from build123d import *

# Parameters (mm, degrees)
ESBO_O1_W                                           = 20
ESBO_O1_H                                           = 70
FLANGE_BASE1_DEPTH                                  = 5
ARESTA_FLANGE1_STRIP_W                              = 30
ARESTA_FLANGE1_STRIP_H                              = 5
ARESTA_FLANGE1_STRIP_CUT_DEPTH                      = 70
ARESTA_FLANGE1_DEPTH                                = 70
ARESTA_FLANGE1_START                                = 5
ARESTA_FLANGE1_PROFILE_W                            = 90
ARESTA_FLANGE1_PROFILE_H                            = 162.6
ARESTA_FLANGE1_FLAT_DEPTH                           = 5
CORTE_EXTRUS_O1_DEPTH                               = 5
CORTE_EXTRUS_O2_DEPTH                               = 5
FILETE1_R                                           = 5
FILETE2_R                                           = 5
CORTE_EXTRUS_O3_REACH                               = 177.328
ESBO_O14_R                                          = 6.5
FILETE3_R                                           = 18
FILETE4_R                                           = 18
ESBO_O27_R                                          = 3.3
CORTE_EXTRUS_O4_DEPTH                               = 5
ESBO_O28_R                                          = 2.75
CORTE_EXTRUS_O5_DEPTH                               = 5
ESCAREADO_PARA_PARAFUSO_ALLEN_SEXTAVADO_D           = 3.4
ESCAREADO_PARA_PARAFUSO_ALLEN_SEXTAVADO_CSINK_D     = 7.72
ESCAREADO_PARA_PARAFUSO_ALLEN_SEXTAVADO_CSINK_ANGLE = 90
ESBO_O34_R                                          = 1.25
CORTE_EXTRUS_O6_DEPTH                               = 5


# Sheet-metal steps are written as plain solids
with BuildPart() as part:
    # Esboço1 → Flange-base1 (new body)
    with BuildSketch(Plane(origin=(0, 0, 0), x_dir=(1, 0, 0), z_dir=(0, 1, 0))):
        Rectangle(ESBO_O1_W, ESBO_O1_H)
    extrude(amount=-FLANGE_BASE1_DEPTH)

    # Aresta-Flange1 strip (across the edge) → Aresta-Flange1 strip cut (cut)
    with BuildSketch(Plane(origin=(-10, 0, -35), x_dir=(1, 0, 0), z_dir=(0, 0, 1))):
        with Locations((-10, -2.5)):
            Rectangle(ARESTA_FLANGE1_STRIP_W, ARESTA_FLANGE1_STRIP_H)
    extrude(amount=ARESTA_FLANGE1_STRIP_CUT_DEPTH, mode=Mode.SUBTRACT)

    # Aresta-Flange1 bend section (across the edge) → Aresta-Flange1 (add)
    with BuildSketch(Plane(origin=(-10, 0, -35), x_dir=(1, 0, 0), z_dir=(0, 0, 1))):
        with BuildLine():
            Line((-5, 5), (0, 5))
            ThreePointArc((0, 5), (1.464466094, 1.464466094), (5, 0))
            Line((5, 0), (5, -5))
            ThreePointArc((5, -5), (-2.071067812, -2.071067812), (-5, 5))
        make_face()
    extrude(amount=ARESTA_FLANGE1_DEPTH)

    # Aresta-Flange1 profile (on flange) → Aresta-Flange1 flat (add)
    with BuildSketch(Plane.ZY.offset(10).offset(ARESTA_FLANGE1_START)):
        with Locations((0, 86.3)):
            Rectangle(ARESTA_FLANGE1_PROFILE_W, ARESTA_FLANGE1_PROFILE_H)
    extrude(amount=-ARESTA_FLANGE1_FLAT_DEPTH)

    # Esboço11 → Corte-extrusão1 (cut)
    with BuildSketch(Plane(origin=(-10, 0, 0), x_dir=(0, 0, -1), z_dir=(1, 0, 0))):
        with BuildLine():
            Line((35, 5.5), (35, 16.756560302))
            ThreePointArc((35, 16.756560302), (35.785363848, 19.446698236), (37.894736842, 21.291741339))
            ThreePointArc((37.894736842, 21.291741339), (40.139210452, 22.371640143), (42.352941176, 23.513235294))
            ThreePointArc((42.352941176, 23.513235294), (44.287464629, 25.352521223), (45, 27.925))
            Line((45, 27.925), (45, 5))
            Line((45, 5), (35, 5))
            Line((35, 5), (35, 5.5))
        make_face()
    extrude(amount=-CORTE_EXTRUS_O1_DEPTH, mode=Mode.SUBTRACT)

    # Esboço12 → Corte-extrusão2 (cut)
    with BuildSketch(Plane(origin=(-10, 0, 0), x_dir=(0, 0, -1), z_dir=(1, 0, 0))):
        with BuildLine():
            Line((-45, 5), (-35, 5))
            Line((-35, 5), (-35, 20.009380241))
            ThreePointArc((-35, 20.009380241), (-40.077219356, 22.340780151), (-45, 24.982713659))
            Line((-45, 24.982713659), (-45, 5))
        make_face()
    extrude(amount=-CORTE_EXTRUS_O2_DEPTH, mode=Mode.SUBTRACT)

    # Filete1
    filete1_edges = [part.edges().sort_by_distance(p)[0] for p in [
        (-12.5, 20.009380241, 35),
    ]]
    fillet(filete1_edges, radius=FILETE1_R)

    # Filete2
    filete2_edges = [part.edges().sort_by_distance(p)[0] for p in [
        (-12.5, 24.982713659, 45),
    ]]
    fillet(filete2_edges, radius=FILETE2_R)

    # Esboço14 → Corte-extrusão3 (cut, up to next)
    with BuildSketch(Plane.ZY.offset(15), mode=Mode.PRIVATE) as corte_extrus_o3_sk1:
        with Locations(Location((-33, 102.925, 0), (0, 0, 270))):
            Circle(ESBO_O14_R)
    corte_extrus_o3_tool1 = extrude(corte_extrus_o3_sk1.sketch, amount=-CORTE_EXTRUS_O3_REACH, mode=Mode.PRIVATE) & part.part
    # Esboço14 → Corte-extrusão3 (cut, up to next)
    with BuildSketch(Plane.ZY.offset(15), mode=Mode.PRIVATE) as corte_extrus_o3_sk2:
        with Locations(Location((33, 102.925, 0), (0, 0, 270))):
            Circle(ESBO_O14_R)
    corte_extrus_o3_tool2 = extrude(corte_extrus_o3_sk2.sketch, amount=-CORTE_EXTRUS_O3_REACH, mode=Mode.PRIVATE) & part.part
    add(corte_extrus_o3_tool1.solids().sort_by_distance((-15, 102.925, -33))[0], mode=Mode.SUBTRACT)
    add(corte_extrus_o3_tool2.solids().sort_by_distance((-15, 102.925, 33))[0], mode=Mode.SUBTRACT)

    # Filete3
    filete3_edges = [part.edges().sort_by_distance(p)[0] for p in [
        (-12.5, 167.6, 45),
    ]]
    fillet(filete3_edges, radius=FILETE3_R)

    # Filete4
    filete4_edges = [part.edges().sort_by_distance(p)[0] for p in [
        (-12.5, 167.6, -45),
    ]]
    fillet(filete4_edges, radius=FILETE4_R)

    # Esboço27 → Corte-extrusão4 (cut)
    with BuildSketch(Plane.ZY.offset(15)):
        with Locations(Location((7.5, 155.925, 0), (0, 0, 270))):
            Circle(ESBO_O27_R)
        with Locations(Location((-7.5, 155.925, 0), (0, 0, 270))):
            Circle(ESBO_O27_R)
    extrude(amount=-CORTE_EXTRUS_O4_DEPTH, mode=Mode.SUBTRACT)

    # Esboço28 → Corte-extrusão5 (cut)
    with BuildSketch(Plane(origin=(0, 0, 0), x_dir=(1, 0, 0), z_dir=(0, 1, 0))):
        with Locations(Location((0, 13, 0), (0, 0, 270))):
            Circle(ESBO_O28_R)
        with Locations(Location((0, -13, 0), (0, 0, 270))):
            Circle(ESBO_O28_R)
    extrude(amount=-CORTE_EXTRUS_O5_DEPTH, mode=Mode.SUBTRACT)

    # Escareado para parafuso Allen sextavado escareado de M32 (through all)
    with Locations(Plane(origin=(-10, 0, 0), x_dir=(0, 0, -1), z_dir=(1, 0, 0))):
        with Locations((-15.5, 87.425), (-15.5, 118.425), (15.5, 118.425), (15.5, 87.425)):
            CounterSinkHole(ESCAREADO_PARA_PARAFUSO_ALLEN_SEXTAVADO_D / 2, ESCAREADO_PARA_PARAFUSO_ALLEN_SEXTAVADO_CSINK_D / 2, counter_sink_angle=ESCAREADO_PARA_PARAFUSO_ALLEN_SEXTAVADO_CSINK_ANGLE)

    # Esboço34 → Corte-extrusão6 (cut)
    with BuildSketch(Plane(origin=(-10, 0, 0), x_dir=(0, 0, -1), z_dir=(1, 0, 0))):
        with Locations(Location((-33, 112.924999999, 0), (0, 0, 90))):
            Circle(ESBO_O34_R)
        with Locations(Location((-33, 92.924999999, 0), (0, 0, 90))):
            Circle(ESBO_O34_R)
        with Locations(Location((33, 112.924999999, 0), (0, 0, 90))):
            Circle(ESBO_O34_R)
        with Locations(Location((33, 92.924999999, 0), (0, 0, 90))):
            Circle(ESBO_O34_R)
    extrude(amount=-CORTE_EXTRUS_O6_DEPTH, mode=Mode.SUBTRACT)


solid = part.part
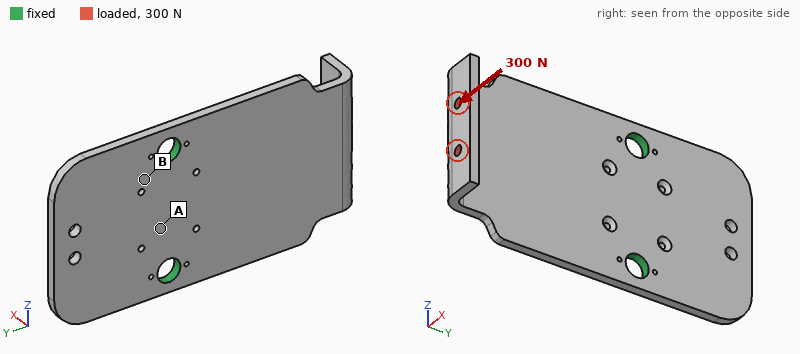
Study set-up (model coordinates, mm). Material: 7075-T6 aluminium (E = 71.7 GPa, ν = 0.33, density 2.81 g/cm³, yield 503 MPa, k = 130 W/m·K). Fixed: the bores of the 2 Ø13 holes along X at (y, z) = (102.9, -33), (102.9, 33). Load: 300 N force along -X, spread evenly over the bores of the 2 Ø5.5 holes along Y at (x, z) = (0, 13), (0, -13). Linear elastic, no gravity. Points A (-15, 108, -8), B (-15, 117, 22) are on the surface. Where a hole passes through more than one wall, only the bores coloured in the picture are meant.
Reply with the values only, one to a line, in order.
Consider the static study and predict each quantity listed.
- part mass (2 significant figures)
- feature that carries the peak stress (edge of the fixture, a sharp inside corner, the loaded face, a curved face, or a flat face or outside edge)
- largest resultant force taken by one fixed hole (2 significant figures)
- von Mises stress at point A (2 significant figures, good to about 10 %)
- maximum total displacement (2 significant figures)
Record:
220 g
a curved face
150 N
21 MPa
1.8 mm
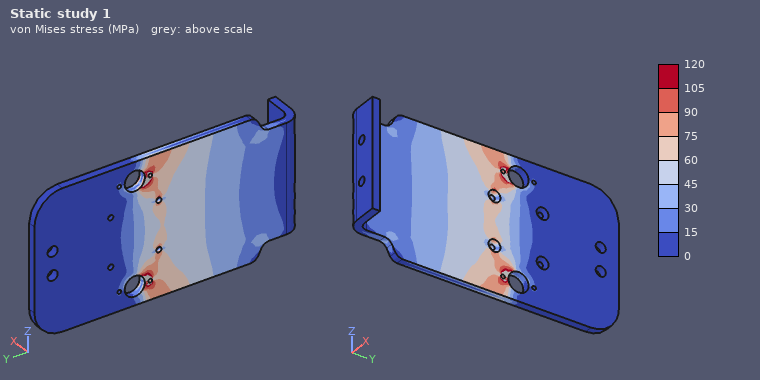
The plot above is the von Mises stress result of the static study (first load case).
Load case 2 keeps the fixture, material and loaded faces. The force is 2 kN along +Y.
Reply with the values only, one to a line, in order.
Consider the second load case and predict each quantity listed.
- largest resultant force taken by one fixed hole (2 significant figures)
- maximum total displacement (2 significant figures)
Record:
1.0 kN
2.3 mm
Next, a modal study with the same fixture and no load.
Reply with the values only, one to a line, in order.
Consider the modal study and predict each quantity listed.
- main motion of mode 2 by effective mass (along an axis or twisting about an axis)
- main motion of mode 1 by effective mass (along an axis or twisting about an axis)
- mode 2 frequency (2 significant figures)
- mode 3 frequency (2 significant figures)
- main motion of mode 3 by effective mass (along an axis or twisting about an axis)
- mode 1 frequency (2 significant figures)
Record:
twisting about Y
along X
1000 Hz
1100 Hz
along X
320 Hz
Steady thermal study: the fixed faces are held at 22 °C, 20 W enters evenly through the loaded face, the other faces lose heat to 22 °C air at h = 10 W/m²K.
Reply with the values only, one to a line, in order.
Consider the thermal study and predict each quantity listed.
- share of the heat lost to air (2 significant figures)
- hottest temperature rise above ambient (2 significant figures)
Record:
21 %
41 K
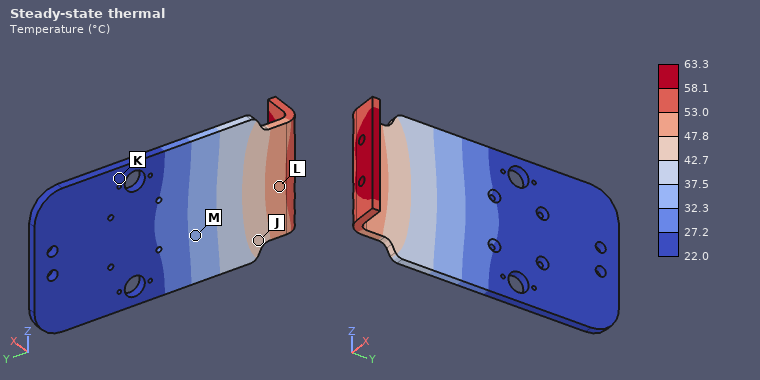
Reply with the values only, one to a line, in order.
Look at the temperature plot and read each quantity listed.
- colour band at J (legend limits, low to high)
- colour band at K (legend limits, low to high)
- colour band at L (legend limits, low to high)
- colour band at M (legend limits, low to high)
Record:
42.7 to 47.8 °C
22.0 to 27.2 °C
47.8 to 53.0 °C
32.3 to 37.5 °C
